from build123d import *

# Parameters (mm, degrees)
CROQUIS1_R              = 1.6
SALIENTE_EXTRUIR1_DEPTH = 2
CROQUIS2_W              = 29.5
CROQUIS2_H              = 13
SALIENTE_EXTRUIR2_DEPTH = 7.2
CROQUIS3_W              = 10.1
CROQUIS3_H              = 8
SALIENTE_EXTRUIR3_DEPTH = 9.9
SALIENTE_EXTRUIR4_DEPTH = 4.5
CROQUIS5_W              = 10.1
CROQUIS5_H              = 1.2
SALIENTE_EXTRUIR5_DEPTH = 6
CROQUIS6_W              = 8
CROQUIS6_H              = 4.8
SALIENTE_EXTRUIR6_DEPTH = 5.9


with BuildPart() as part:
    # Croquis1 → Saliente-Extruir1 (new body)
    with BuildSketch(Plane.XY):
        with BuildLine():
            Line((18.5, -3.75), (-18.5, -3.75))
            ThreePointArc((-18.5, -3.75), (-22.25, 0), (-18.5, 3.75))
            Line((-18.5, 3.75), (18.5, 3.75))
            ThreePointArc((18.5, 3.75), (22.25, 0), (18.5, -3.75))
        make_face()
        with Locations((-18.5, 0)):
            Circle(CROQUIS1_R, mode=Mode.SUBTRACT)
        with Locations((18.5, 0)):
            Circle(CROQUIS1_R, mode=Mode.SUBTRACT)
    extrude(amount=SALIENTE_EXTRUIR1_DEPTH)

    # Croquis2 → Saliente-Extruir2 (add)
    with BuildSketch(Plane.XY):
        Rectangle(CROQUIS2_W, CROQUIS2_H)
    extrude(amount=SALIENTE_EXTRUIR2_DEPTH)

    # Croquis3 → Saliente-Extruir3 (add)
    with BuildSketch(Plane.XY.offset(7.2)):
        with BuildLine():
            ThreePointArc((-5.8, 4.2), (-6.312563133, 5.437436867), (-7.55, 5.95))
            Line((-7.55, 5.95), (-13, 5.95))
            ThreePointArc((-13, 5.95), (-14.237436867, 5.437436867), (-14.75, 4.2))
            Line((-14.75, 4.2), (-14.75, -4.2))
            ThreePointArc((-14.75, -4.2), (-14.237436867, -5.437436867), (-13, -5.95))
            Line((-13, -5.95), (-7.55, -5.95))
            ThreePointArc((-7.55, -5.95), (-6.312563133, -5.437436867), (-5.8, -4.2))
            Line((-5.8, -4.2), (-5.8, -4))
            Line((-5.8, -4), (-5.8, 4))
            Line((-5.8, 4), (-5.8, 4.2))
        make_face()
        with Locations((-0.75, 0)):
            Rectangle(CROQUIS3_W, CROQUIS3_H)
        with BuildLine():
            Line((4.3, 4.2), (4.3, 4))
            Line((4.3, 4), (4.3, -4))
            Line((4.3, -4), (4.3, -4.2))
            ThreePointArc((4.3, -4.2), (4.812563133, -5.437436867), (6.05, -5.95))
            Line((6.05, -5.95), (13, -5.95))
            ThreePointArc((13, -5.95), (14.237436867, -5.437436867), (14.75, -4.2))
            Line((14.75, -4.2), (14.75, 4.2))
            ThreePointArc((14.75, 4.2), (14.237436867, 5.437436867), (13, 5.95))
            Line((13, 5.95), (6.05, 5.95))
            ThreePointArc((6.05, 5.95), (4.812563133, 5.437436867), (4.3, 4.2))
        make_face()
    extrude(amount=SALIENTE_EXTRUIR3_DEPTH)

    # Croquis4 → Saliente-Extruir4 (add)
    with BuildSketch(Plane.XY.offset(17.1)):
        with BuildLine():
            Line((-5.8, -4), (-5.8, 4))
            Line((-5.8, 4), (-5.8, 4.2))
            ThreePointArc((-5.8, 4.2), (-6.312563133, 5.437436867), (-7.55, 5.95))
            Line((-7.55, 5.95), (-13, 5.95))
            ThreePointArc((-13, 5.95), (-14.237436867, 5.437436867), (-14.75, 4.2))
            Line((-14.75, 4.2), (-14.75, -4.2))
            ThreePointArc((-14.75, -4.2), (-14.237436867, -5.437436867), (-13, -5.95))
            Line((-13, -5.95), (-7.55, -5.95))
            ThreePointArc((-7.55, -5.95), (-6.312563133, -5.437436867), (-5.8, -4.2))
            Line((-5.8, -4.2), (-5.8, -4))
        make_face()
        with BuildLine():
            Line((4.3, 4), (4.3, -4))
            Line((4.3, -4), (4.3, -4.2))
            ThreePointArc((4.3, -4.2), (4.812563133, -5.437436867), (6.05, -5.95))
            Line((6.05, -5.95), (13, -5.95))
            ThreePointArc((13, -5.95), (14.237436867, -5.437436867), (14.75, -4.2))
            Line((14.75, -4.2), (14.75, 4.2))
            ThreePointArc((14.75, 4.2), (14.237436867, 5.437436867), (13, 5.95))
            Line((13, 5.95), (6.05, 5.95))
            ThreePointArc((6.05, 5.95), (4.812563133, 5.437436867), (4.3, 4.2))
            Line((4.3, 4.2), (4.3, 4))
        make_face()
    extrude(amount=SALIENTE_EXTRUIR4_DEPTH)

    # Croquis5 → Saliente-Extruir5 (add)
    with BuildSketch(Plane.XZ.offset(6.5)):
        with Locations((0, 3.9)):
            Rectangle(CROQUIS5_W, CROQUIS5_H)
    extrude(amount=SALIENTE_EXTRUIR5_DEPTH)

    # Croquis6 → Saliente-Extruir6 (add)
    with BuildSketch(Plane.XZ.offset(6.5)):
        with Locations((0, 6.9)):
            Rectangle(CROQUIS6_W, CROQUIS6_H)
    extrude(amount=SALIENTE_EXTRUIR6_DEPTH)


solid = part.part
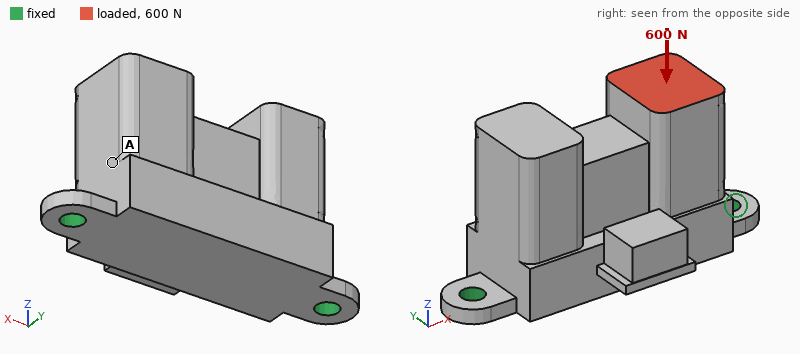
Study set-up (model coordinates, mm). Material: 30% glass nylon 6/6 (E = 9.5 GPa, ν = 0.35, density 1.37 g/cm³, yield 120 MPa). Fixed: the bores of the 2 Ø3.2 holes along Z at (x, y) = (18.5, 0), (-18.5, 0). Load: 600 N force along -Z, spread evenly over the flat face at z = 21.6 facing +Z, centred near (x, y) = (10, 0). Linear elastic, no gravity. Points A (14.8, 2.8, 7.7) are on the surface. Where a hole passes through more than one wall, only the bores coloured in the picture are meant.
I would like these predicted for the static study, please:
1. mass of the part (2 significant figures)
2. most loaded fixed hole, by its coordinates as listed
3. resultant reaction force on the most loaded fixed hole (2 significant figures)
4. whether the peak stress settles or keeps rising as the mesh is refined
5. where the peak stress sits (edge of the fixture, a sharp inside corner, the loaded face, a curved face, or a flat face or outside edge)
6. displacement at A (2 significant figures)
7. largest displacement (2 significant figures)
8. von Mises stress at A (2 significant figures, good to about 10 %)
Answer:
10.0 g
(18.5, 0)
510 N
keeps rising
edge of the fixture
0.087 mm
0.10 mm
12 MPa
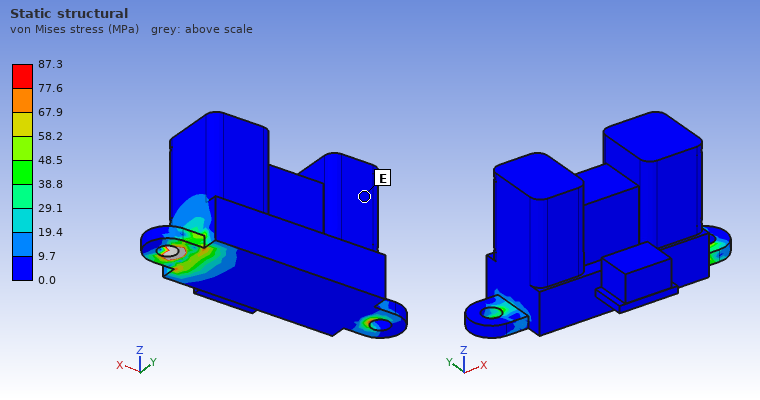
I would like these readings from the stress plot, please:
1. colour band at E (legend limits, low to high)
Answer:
0.0 to 9.7 MPa
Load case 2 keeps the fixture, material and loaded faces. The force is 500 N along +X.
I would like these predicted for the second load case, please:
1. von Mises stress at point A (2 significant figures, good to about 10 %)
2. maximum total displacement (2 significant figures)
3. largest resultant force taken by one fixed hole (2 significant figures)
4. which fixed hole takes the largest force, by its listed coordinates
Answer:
11 MPa
0.13 mm
440 N
(-18.5, 0)
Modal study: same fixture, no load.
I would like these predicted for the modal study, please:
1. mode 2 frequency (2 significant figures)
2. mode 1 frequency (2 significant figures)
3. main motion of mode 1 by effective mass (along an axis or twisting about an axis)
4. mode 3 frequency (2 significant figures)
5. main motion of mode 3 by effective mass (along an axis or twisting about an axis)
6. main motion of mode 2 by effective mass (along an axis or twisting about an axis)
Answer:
5200 Hz
1100 Hz
along Y
6000 Hz
along X
along Z
